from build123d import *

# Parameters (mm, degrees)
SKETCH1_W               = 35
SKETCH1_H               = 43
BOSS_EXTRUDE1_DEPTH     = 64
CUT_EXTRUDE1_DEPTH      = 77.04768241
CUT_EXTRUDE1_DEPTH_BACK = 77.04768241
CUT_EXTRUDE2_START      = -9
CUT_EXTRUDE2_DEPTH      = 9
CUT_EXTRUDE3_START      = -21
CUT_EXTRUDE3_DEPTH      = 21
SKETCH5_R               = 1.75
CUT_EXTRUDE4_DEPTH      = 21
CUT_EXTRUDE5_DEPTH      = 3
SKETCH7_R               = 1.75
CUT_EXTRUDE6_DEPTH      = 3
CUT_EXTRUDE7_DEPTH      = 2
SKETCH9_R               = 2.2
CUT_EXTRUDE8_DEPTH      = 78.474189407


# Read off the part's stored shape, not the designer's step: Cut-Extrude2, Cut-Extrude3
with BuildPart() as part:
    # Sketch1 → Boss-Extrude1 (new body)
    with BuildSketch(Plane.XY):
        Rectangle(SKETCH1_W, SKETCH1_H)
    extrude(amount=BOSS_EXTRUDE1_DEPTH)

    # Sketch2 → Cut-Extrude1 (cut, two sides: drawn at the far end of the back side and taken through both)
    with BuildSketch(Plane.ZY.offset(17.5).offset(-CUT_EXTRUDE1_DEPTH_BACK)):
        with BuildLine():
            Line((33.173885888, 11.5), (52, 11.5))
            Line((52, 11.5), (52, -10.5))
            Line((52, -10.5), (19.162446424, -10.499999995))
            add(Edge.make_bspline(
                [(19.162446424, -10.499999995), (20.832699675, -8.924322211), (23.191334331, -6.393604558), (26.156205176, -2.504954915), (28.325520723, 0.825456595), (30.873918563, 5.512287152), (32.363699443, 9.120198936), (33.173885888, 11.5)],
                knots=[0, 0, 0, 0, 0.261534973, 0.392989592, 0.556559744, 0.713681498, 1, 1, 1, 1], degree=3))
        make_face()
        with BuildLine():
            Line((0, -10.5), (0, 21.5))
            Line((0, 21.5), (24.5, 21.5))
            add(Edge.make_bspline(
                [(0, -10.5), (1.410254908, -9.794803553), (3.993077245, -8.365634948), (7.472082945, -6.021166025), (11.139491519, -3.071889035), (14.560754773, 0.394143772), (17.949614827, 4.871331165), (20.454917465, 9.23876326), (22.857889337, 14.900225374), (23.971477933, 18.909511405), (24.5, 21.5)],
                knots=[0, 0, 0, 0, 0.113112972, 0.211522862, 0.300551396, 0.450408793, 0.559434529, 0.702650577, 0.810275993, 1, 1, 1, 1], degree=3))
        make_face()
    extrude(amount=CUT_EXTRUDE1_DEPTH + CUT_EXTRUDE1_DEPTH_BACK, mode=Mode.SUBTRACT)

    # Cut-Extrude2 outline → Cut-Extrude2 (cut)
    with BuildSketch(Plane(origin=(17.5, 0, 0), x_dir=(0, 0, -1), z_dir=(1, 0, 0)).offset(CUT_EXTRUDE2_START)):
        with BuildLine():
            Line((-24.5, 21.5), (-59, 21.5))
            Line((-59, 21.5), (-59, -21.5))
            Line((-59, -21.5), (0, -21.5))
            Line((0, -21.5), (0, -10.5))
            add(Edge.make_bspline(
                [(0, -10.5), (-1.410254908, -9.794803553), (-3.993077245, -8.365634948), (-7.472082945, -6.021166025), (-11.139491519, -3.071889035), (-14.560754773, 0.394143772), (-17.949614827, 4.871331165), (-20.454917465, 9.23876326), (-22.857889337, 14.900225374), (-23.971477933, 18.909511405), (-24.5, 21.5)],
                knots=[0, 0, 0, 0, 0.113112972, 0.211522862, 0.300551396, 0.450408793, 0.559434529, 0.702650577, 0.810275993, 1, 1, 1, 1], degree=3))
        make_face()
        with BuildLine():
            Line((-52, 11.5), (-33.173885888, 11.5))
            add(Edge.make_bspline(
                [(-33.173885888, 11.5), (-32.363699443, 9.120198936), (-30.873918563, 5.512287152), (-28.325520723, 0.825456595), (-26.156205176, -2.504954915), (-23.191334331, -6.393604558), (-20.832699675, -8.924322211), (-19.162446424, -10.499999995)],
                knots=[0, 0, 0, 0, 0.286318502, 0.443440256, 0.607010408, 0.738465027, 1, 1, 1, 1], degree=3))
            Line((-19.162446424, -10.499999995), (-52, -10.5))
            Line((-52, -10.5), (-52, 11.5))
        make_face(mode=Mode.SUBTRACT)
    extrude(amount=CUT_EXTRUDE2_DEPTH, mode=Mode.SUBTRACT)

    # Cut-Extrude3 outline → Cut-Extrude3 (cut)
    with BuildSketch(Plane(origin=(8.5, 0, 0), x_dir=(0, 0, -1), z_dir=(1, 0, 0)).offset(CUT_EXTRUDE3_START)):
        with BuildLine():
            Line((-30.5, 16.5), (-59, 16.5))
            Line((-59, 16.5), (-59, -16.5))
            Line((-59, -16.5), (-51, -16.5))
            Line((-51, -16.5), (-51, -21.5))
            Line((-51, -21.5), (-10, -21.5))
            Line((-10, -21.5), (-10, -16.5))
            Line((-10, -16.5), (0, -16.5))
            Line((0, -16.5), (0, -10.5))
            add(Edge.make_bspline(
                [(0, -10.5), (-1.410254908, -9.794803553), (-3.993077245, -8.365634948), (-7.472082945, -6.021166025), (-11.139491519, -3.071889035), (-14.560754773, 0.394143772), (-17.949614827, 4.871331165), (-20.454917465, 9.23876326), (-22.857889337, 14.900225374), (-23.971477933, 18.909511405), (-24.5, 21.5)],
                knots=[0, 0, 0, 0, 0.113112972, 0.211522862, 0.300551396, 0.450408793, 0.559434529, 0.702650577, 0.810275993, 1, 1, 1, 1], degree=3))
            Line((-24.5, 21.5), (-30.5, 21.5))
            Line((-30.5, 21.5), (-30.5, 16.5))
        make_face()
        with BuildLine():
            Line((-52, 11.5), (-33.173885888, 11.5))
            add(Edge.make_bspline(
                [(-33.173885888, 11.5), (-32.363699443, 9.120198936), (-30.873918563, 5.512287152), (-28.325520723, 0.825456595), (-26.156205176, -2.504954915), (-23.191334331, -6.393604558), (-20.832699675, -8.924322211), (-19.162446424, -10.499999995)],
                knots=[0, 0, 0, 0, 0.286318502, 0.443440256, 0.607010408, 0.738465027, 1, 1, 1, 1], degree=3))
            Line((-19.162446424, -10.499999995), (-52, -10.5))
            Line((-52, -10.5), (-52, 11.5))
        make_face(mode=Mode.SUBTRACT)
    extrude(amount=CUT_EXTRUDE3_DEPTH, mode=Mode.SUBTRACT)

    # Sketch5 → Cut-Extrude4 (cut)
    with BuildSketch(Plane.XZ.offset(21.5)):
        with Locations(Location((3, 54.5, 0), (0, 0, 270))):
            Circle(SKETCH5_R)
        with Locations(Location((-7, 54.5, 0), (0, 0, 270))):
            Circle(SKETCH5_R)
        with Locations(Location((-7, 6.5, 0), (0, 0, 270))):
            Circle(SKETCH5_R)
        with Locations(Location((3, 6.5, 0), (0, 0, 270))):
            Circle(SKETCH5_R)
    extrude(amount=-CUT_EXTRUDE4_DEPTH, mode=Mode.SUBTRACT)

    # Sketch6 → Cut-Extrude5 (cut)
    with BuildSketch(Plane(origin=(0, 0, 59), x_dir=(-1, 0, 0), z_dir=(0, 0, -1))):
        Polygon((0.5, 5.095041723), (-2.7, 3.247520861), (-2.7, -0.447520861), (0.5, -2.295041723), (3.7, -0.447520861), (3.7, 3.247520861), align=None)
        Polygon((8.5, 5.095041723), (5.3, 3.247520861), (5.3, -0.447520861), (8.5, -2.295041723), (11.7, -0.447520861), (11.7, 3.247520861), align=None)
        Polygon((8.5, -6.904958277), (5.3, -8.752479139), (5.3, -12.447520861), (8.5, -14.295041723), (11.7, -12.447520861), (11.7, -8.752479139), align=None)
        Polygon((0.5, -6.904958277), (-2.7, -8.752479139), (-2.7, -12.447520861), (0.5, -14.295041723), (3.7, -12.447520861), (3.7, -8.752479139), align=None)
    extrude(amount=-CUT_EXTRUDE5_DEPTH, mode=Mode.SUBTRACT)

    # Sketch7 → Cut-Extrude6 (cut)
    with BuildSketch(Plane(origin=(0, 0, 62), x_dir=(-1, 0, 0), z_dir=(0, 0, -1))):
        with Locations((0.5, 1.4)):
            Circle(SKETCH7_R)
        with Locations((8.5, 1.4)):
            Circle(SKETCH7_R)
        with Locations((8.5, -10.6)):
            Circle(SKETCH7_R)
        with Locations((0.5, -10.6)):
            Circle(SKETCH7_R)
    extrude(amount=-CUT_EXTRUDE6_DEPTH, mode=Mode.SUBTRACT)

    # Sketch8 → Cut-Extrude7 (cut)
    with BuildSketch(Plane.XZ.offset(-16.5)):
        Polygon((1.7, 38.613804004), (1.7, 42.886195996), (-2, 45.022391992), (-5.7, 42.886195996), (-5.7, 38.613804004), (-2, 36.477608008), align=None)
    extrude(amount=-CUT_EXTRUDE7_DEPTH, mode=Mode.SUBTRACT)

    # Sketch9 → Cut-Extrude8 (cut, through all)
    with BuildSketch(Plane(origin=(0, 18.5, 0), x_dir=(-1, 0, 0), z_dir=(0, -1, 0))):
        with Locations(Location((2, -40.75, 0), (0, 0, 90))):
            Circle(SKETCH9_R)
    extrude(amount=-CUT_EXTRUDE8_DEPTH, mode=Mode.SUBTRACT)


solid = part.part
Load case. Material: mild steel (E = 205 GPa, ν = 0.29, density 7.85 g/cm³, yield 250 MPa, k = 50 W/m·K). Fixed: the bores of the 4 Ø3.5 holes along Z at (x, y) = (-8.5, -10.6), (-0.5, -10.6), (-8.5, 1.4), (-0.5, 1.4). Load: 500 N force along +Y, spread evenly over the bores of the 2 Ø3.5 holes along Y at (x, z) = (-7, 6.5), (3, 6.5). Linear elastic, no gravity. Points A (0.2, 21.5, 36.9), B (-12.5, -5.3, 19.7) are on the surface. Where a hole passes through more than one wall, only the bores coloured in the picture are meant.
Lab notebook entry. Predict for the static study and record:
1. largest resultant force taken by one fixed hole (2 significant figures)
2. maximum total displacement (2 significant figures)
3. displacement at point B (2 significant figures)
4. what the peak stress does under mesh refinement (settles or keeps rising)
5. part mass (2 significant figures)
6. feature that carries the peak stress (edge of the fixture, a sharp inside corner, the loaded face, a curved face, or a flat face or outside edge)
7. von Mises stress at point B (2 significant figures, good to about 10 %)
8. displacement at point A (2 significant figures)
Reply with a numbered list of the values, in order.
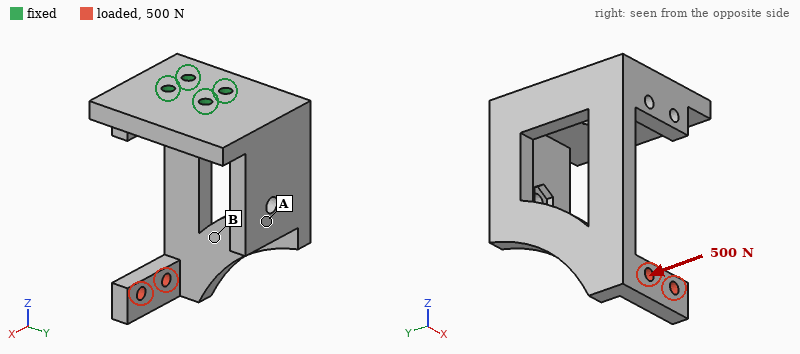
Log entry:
1. 1.7 kN
2. 0.29 mm
3. 0.074 mm
4. keeps rising
5. 150 g
6. edge of the fixture
7. 71 MPa
8. 0.055 mm
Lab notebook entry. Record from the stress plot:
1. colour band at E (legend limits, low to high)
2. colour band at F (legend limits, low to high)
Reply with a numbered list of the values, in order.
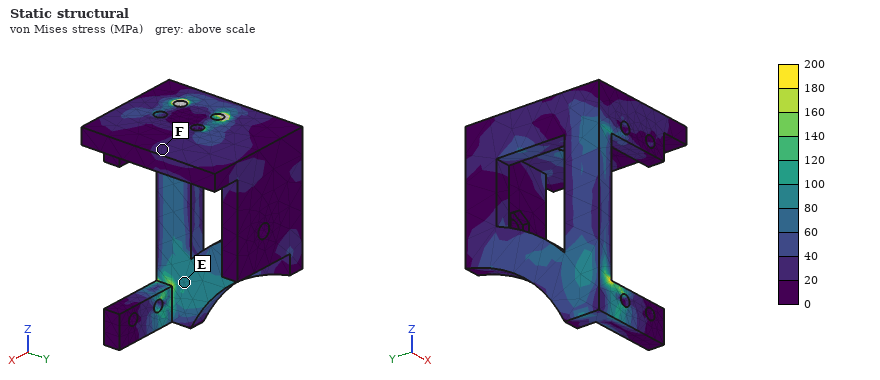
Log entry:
1. 80 to 100 MPa
2. 20 to 40 MPa
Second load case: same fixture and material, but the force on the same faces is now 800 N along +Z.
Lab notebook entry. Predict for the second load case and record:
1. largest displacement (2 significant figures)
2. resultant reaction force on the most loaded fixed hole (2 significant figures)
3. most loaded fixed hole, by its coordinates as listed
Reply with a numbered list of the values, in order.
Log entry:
1. 0.42 mm
2. 910 N
3. (-8.5, -10.6)
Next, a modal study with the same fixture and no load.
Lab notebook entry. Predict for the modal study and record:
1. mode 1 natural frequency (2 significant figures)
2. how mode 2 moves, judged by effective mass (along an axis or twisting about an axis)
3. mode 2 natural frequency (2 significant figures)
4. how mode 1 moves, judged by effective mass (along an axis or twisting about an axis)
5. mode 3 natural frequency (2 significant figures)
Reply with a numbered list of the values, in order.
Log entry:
1. 1100 Hz
2. along Y
3. 1900 Hz
4. along X
5. 3200 Hz
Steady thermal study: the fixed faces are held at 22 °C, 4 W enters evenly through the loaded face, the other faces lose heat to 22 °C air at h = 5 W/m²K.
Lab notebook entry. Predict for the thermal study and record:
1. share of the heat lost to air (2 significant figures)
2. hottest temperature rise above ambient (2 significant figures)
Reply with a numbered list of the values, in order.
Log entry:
1. 16 %
2. 64 K
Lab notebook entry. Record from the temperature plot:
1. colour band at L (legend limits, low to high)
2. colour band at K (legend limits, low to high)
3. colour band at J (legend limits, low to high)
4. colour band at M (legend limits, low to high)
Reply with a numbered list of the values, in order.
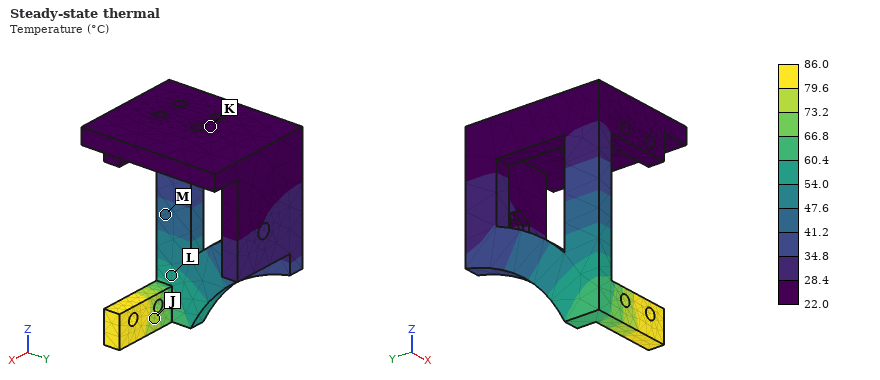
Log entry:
1. 54.0 to 60.4 °C
2. 22.0 to 28.4 °C
3. 73.2 to 79.6 °C
4. 41.2 to 47.6 °C
